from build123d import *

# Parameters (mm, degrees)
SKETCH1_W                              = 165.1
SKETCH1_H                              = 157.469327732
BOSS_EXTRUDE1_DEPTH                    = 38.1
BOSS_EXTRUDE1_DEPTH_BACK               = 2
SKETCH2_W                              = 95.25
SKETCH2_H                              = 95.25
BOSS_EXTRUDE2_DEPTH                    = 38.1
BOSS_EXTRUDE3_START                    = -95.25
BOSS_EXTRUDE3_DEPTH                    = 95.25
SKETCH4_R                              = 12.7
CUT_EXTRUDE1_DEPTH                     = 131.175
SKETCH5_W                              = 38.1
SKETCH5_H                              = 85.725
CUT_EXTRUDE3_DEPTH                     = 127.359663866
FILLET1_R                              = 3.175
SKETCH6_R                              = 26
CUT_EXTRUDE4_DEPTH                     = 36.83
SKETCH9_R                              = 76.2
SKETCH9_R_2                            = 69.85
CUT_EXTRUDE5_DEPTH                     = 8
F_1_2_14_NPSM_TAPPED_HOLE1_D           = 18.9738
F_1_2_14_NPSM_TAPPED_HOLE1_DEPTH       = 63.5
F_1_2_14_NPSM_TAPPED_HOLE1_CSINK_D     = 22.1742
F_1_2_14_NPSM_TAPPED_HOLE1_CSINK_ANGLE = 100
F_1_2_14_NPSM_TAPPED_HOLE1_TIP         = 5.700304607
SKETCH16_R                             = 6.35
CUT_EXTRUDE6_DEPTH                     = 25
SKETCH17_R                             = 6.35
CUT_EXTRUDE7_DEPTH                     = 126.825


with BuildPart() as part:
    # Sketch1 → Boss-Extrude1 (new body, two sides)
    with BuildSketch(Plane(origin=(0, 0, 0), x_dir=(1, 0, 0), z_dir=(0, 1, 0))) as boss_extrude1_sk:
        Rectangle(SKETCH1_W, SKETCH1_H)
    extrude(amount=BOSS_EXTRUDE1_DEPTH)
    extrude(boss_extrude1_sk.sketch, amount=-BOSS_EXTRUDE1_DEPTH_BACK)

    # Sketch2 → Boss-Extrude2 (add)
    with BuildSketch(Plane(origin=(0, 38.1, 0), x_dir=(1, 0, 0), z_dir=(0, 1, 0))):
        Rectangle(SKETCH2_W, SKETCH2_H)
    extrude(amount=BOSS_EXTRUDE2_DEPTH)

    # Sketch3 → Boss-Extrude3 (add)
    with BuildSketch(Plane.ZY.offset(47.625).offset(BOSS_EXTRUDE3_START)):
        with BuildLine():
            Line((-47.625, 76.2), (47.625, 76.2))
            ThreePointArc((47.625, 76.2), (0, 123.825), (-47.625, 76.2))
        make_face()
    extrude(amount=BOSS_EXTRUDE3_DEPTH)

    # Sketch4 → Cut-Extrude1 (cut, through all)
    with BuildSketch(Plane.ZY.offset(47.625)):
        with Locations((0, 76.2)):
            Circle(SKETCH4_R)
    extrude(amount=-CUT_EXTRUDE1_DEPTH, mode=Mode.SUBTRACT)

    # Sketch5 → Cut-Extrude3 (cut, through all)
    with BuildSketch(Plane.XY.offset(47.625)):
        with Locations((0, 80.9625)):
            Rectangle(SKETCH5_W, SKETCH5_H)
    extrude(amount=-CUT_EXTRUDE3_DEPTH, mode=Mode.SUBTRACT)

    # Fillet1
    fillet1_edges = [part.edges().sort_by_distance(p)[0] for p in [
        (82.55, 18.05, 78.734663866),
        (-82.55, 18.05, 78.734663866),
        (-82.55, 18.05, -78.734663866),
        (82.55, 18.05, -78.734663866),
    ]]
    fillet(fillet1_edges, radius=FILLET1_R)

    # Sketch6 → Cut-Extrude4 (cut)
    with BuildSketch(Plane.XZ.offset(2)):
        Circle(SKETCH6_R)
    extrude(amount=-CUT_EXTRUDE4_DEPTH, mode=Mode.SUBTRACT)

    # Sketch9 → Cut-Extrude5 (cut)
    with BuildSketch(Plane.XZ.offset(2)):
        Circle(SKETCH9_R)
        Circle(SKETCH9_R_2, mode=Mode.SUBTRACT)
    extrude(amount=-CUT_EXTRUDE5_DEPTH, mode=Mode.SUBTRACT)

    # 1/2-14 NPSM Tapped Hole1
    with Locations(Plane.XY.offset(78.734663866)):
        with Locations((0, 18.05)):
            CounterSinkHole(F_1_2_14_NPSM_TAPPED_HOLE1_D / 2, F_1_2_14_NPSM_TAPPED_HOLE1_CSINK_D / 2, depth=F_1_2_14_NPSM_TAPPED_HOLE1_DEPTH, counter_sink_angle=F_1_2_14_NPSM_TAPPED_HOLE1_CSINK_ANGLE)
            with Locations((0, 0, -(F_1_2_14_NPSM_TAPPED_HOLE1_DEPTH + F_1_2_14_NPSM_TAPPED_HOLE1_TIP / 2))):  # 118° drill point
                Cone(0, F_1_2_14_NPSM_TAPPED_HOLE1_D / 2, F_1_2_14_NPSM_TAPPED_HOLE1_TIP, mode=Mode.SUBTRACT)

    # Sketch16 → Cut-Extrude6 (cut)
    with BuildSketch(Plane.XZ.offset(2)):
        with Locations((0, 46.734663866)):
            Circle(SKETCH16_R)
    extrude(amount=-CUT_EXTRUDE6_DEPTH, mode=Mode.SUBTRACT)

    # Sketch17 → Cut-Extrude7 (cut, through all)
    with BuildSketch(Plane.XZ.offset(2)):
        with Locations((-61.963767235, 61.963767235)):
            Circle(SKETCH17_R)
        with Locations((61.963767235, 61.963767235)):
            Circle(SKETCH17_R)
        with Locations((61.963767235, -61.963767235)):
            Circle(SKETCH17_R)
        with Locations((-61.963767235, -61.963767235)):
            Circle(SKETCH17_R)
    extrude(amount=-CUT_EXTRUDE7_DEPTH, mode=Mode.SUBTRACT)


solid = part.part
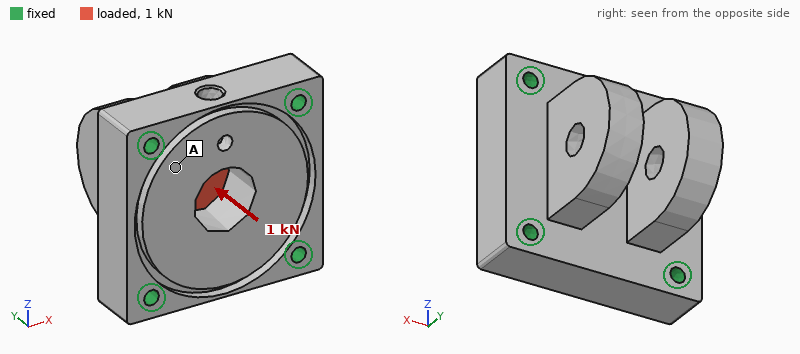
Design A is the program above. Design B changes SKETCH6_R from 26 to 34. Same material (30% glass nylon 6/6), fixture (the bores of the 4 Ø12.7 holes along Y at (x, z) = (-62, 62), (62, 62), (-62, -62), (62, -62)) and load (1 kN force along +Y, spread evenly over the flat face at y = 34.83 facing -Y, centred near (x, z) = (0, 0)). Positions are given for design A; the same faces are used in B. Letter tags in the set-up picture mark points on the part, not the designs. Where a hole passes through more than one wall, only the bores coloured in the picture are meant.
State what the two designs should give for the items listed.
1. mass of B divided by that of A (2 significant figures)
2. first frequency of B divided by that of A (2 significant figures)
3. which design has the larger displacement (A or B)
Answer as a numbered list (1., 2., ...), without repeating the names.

1. 0.96
2. 0.94
3. A
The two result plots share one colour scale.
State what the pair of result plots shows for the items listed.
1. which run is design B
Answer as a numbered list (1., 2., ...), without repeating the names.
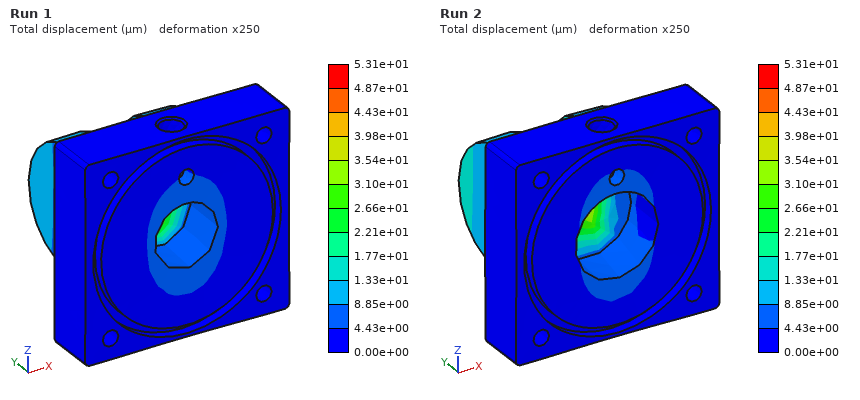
1. Run 2
